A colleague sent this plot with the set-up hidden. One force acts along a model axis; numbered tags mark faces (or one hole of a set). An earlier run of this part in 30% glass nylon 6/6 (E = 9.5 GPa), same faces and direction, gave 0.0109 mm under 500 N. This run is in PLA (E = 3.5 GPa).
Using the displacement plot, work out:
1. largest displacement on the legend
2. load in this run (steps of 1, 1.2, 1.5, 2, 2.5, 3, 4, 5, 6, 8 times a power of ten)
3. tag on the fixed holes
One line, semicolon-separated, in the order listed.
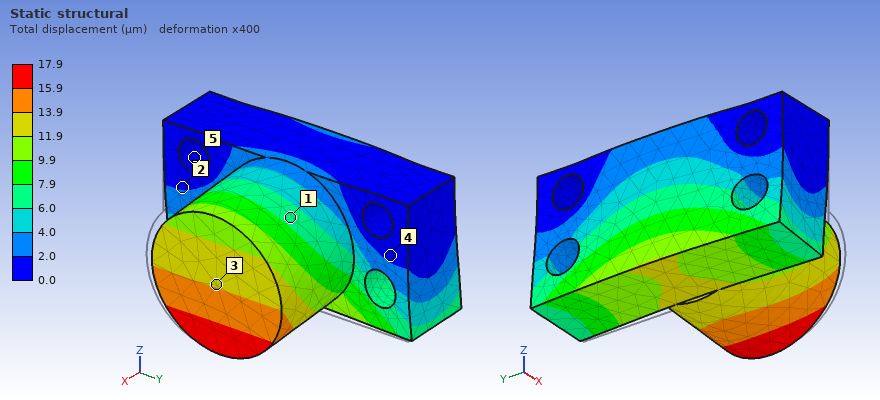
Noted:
17.9 µm; 300 N; 5
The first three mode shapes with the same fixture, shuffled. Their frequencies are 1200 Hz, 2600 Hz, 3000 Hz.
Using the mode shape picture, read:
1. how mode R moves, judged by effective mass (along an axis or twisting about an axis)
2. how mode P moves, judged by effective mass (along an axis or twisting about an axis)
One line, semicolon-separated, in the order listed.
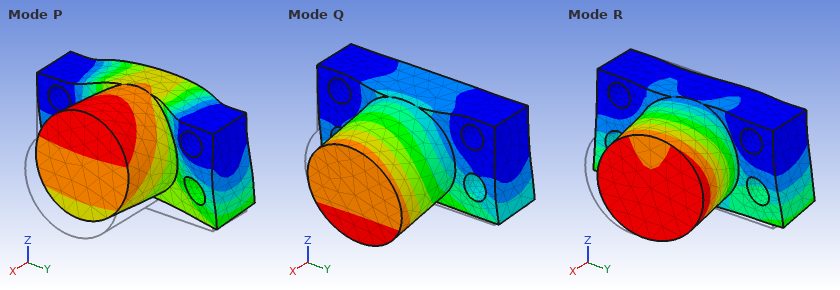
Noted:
along Y; along X
